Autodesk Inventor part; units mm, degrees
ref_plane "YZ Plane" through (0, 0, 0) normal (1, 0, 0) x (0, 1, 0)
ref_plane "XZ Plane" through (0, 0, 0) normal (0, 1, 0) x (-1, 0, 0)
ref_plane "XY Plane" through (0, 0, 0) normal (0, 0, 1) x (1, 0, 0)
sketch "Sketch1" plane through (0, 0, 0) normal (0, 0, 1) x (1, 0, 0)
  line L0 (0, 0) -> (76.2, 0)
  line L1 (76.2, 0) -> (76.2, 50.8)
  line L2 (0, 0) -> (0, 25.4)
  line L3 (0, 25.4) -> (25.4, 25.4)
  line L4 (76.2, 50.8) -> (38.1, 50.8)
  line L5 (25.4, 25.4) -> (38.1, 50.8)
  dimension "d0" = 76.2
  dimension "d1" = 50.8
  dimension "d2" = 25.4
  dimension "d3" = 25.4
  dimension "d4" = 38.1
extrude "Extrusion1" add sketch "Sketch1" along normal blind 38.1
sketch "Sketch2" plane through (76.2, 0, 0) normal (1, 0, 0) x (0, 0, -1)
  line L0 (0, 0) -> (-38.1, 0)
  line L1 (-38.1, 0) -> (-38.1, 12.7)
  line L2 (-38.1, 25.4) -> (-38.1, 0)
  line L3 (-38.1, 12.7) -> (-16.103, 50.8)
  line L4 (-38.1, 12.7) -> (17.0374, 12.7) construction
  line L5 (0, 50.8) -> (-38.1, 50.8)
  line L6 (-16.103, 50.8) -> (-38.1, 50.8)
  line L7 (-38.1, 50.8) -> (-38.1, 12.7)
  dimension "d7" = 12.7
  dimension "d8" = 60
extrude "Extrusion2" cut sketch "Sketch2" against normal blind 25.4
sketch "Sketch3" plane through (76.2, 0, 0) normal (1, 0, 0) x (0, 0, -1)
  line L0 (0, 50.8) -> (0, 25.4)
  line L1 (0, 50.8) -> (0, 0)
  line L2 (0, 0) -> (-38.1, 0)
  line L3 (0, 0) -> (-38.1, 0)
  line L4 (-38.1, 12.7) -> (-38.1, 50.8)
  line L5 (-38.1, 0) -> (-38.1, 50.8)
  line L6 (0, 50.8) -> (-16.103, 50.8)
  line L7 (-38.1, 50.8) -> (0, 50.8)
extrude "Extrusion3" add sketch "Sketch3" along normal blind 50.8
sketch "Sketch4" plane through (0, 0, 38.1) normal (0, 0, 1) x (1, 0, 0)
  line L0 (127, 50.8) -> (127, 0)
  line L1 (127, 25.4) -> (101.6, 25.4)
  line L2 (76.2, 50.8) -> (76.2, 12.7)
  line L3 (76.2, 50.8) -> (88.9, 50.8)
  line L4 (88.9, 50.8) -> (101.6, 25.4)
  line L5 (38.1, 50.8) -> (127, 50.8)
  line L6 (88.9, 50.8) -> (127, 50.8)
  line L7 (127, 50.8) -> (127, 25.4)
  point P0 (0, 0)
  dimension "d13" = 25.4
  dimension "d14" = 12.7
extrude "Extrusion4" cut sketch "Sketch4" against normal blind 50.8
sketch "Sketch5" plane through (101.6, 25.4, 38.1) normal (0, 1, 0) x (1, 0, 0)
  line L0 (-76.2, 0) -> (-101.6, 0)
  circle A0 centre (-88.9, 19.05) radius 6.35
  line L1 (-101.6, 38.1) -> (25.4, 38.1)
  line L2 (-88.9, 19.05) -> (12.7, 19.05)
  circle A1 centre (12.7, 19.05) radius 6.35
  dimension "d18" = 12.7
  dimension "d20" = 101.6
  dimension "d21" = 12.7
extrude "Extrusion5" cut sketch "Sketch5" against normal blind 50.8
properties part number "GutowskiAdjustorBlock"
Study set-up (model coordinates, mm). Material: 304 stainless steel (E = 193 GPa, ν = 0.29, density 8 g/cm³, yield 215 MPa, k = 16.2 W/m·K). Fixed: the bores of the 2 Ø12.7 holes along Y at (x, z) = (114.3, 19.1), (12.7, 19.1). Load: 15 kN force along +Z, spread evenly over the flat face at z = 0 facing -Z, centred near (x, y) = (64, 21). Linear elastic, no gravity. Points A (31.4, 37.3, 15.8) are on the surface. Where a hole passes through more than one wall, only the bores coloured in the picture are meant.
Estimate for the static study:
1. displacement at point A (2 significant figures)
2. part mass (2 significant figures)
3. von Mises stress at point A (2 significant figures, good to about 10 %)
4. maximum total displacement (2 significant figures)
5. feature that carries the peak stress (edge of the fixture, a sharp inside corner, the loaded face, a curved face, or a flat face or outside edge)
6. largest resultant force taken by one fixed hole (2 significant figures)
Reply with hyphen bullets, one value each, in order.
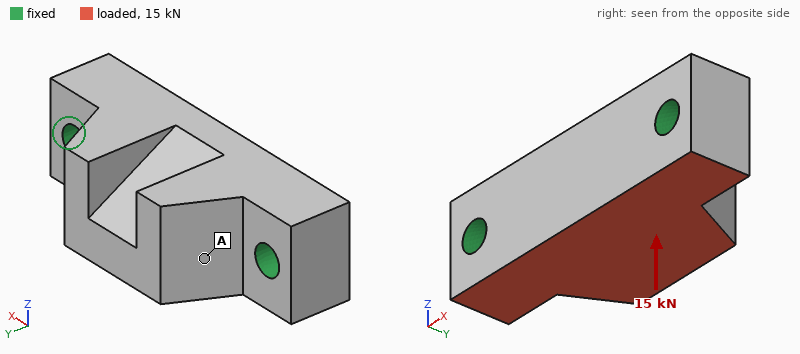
- 6.3 µm
- 1.3 kg
- 9.7 MPa
- 11 µm
- edge of the fixture
- 7.5 kN
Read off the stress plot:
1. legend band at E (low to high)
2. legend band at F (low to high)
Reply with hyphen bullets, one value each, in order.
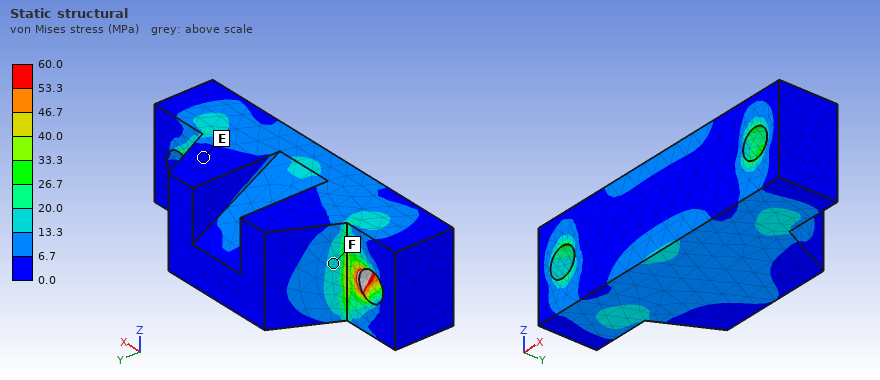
- 0.0 to 6.7 MPa
- 13.3 to 20.0 MPa
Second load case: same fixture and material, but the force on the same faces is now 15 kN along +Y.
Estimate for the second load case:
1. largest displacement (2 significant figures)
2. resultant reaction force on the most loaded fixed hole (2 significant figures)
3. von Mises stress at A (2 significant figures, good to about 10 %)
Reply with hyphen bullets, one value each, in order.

- 15 µm
- 7.7 kN
- 9.7 MPa
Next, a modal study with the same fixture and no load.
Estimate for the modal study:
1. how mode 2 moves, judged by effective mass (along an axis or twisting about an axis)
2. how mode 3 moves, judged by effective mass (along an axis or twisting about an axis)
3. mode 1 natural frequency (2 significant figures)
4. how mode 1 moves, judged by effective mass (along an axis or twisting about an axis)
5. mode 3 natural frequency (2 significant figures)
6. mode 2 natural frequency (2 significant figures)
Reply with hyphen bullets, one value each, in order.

- along Y
- along Z
- 6400 Hz
- along Z
- 11 kHz
- 9400 Hz
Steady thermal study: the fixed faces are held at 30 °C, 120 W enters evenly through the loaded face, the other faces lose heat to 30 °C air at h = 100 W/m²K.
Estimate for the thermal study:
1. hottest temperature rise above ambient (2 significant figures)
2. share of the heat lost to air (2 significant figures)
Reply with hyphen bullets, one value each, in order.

- 70 K
- 37 %
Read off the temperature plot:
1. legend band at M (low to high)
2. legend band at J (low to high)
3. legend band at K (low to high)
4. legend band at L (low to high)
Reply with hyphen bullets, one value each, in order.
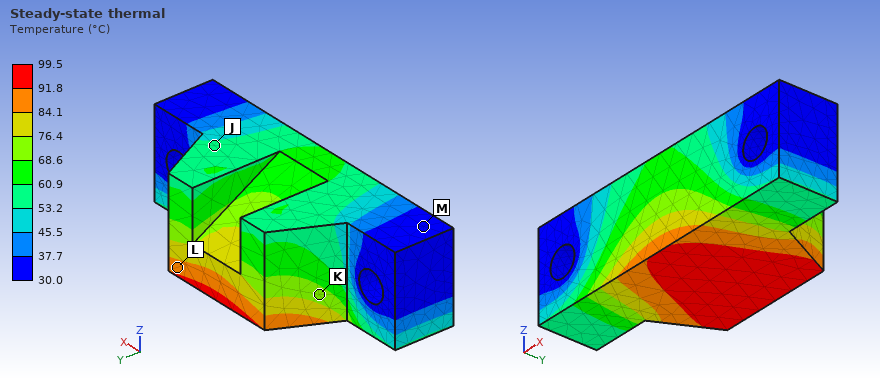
- 30.0 to 37.7 °C
- 53.2 to 60.9 °C
- 68.6 to 76.4 °C
- 84.1 to 91.8 °C
